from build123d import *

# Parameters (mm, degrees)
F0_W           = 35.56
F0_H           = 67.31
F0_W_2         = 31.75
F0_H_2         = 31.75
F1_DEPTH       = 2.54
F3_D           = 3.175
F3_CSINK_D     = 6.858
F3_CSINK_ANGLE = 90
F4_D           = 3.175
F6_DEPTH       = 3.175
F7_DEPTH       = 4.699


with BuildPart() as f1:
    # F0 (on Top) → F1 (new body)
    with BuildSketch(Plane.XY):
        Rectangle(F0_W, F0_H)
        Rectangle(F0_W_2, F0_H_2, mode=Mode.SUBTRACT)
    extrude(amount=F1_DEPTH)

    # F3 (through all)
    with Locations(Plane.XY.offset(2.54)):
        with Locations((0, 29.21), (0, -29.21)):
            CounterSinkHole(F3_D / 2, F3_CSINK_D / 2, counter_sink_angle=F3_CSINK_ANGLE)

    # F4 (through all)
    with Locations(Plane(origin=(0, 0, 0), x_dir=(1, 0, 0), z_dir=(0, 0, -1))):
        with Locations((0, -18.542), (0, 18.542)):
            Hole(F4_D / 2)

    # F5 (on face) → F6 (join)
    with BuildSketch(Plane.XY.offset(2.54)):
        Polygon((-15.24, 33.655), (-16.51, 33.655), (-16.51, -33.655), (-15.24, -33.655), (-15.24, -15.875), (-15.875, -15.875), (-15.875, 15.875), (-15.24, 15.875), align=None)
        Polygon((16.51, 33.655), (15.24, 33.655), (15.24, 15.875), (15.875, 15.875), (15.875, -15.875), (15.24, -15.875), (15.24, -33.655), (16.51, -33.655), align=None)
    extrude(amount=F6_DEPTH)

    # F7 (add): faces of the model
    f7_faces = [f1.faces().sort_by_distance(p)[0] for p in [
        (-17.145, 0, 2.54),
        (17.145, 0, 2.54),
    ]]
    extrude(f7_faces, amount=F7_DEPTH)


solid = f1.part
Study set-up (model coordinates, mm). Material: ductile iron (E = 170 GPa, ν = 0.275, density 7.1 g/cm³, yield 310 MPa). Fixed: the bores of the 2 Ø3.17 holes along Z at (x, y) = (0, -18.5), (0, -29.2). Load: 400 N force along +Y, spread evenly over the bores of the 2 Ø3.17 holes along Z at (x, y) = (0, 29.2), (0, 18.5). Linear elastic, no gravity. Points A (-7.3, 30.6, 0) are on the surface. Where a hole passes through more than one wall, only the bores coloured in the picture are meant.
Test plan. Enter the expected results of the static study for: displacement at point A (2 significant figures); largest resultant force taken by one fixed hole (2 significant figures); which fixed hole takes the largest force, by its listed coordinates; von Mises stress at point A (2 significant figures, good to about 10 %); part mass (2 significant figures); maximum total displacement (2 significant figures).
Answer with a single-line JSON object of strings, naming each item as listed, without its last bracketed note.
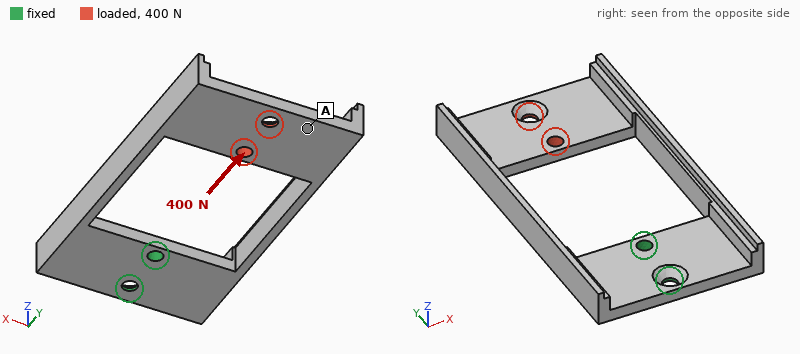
{"displacement at point A": "74 µm", "largest resultant force taken by one fixed hole": "230 N", "which fixed hole takes the largest force, by its listed coordinates": "(0, -18.5)", "von Mises stress at point A": "15 MPa", "part mass": "33 g", "maximum total displacement": "82 µm"}
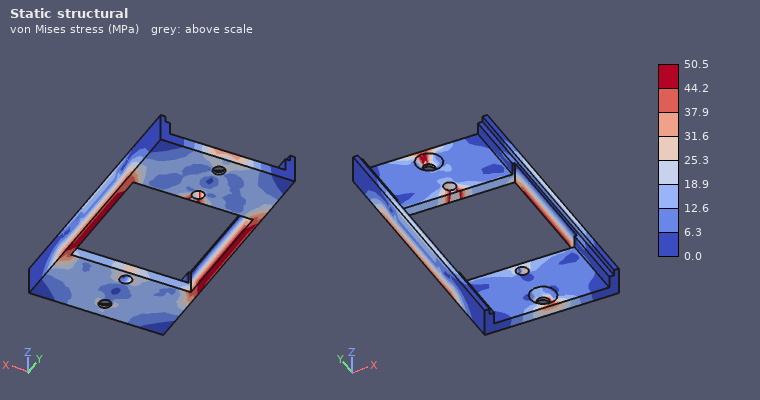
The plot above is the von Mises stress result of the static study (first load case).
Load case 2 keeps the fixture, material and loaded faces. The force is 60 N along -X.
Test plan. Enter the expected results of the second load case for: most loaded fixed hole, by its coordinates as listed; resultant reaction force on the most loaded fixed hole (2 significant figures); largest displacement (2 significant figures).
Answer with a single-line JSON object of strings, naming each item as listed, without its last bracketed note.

{"most loaded fixed hole, by its coordinates as listed": "(0, -18.5)", "resultant reaction force on the most loaded fixed hole": "250 N", "largest displacement": "0.18 mm"}
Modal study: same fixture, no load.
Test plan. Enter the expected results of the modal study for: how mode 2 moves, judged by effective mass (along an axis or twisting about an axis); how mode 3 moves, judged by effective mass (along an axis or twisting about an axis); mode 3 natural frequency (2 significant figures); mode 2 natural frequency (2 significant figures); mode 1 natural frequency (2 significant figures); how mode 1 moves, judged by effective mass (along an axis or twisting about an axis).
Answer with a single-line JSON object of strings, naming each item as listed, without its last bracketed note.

{"how mode 2 moves, judged by effective mass": "along X", "how mode 3 moves, judged by effective mass": "twisting about Y", "mode 3 natural frequency": "1300 Hz", "mode 2 natural frequency": "750 Hz", "mode 1 natural frequency": "650 Hz", "how mode 1 moves, judged by effective mass": "along Z"}
